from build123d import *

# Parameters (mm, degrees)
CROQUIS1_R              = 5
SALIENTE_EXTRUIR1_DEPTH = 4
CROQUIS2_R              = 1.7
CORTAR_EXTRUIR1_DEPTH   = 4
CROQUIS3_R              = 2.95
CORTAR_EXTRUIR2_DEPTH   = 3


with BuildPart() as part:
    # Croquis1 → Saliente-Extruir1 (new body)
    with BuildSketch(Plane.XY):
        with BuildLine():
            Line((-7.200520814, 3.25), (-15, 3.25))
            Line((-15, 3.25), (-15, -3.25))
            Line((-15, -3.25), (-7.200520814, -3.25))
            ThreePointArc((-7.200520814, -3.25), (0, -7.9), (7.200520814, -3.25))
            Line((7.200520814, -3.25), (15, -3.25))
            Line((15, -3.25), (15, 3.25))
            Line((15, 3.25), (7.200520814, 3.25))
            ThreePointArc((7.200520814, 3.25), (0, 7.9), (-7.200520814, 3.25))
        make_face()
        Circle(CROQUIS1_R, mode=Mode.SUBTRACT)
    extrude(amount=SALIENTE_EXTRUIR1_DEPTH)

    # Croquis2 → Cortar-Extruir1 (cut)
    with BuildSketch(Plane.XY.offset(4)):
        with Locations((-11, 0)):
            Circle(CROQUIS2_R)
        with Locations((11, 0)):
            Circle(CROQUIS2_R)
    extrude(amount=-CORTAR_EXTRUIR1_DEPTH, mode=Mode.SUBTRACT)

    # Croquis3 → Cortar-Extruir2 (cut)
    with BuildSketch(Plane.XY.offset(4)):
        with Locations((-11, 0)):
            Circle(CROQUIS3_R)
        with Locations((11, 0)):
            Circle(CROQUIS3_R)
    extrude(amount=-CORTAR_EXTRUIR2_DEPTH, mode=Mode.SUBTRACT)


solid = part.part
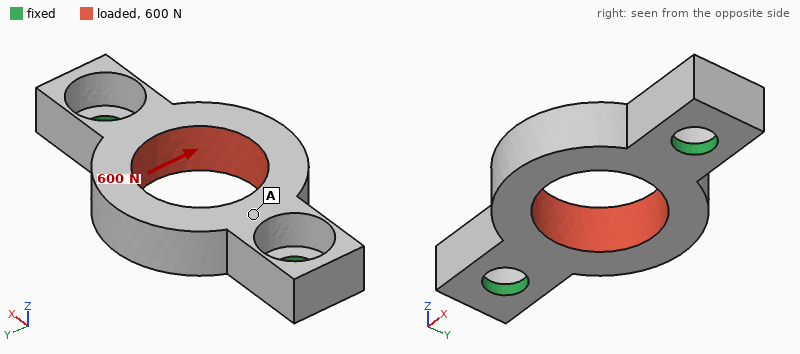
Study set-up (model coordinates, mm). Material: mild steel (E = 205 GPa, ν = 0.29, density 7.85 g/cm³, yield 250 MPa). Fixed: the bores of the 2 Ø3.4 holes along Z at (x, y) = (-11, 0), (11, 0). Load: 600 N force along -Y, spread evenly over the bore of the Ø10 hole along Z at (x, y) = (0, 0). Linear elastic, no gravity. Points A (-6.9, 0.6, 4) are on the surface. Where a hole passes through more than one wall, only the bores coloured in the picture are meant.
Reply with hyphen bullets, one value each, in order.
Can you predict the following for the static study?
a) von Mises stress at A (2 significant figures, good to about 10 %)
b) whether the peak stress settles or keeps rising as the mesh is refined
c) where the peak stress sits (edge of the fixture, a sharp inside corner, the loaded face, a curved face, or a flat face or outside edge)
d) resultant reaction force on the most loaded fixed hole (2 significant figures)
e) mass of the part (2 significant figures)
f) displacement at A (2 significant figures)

- 49 MPa
- keeps rising
- edge of the fixture
- 300 N
- 5.3 g
- 5.2 µm
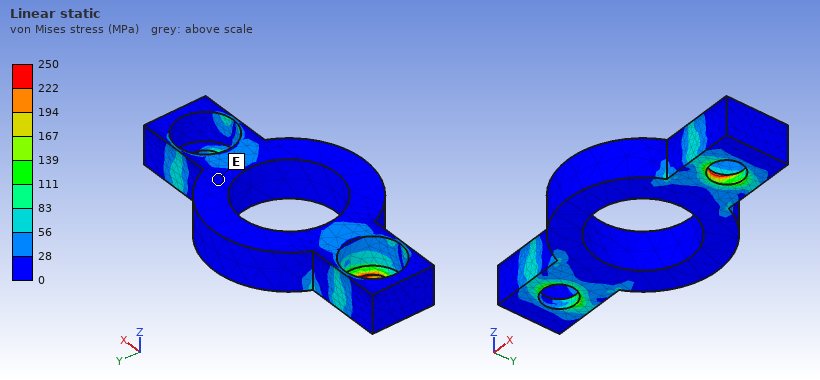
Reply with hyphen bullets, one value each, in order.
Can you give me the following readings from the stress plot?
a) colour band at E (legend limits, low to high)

- 0 to 28 MPa
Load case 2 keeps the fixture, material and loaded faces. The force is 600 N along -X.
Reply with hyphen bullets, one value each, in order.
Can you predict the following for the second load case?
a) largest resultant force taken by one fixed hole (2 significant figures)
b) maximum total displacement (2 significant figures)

- 300 N
- 1.6 µm
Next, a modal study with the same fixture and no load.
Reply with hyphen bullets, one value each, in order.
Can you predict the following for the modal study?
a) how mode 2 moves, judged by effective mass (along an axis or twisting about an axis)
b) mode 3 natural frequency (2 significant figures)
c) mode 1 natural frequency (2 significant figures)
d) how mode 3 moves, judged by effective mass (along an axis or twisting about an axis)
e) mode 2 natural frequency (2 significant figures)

- along Z
- 43 kHz
- 14 kHz
- along Y
- 20 kHz
